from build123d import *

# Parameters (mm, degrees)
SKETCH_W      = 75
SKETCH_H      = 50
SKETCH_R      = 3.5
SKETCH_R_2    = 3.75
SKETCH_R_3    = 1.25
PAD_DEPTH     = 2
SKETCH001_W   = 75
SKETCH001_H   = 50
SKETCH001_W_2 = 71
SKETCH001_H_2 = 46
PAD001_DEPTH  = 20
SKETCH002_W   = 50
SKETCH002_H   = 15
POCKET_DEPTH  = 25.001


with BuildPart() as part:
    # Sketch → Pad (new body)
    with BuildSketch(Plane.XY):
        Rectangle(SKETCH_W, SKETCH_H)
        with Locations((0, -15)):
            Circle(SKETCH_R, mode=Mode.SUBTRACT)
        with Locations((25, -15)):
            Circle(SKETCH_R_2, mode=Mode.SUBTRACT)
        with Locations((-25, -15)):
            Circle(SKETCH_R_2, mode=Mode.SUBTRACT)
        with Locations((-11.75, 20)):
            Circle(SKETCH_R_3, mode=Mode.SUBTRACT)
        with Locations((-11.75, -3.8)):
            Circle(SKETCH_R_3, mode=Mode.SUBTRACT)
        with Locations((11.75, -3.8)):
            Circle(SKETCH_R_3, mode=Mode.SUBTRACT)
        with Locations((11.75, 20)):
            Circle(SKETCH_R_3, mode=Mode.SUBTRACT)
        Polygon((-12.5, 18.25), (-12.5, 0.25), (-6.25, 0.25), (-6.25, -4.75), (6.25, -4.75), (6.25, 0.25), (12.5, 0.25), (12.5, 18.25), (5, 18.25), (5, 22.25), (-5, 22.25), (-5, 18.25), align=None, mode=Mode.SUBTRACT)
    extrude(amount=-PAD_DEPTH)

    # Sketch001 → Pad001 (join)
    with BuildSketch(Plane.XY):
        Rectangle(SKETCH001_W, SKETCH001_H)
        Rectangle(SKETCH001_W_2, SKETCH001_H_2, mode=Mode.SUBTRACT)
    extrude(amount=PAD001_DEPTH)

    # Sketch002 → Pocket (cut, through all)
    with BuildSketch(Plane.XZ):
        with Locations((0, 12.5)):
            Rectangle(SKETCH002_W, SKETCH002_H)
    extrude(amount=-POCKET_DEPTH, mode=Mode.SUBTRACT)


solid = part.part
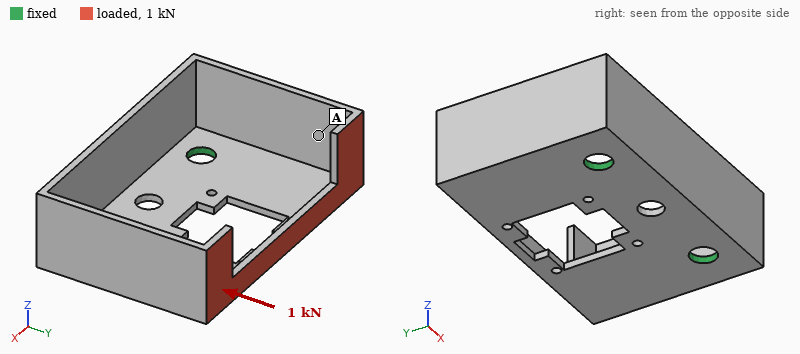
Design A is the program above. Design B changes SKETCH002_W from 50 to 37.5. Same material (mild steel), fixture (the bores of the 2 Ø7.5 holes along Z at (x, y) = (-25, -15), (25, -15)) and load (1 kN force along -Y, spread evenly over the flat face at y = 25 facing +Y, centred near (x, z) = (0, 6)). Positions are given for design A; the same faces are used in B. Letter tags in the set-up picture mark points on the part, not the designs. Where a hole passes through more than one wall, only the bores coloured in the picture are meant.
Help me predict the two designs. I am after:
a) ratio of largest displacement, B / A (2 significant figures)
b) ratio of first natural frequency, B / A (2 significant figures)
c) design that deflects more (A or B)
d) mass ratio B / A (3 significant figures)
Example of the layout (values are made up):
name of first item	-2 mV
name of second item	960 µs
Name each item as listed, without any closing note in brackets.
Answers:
ratio of largest displacement, B / A	1.4
ratio of first natural frequency, B / A	0.96
design that deflects more	B
mass ratio B / A	1.03
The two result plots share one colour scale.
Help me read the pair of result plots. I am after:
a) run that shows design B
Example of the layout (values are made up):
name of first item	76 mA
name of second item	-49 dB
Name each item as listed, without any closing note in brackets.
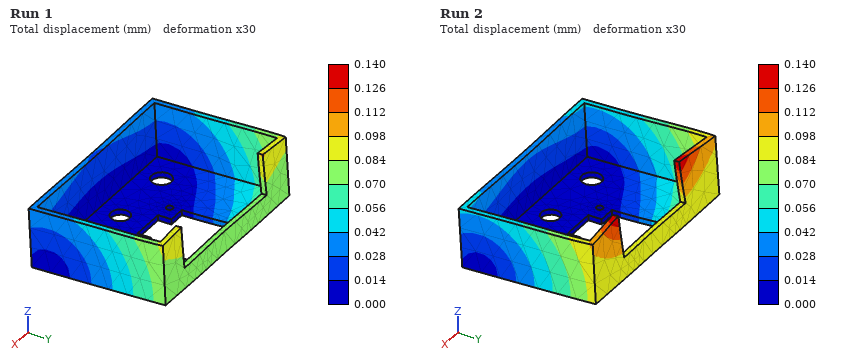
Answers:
run that shows design B	Run 2
